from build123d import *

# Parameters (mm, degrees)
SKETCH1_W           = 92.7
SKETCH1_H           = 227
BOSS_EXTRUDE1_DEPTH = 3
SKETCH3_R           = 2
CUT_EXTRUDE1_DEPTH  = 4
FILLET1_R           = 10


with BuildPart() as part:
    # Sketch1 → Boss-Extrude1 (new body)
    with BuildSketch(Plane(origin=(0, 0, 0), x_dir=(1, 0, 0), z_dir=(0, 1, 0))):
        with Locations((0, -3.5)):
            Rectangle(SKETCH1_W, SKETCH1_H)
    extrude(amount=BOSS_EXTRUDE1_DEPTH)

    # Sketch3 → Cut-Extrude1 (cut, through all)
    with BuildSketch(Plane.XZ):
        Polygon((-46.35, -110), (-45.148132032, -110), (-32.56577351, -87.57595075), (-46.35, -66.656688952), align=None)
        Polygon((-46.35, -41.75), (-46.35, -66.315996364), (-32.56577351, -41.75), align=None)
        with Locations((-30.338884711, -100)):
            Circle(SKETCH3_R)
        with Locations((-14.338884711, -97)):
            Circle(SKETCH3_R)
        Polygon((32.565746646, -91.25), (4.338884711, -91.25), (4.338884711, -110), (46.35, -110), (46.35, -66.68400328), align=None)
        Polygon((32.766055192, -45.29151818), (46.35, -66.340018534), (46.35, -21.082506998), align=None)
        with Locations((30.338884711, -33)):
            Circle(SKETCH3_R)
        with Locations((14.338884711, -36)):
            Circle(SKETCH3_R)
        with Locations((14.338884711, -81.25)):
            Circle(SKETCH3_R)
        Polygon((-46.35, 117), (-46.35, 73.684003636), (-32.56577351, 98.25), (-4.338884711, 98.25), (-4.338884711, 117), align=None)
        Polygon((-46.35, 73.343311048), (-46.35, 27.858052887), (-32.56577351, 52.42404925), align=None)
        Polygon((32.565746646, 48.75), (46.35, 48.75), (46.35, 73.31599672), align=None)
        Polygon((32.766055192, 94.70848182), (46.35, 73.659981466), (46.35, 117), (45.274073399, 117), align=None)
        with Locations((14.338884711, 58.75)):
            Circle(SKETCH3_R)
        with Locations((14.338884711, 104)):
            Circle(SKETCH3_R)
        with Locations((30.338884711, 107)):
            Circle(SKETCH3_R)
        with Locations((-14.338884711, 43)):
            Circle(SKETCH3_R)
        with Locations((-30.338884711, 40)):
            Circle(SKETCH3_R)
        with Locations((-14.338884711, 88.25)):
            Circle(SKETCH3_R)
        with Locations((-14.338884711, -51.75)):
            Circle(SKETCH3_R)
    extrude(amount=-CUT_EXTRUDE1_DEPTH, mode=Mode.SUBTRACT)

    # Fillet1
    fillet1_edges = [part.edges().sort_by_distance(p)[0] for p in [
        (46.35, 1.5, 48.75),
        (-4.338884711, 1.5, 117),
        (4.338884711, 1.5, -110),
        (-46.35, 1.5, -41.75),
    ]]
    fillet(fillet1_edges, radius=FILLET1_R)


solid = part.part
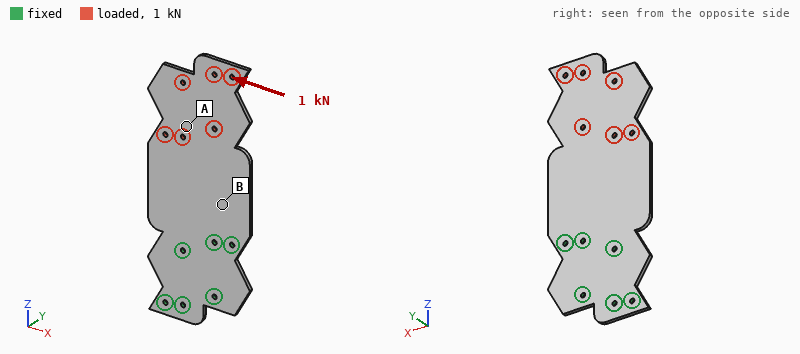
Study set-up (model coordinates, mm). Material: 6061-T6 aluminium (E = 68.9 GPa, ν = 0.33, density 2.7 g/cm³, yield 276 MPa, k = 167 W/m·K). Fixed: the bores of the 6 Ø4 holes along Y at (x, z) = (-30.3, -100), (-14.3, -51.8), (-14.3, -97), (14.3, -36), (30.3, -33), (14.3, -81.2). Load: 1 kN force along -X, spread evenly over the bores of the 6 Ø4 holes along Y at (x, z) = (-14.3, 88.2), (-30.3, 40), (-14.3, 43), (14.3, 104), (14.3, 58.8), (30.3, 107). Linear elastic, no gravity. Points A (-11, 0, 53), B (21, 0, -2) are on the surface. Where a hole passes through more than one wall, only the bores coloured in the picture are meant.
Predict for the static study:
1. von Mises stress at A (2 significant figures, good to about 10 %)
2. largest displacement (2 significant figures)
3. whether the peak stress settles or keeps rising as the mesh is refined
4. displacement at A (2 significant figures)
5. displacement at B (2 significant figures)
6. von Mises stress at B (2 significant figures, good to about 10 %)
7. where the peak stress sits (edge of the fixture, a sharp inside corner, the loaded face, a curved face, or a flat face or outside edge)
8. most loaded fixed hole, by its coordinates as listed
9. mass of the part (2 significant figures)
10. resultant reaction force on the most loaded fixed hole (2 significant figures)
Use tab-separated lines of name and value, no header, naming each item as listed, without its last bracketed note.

von Mises stress at A	6.2 MPa
largest displacement	0.14 mm
whether the peak stress settles or keeps rising as the mesh is refined	keeps rising
displacement at A	0.070 mm
displacement at B	0.024 mm
von Mises stress at B	14 MPa
where the peak stress sits	edge of the fixture
most loaded fixed hole, by its coordinates as listed	(30.3, -33)
mass of the part	140 g
resultant reaction force on the most loaded fixed hole	1.9 kN
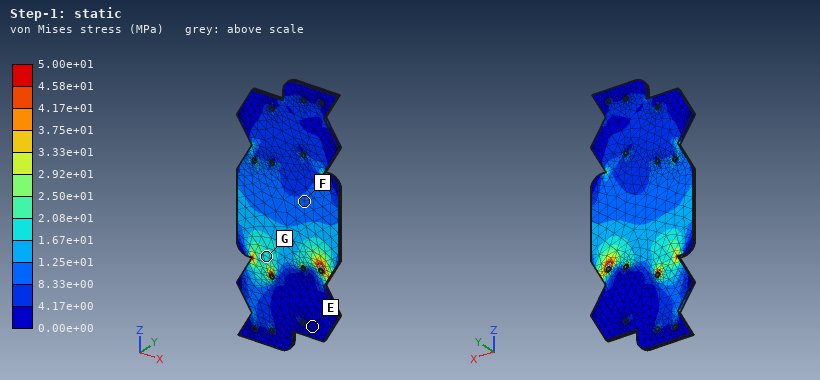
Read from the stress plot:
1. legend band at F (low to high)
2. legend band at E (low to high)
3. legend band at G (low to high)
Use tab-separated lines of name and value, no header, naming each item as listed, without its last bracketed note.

legend band at F	8.33e+00 to 1.25e+01 MPa
legend band at E	0.00e+00 to 4.17e+00 MPa
legend band at G	1.67e+01 to 2.08e+01 MPa
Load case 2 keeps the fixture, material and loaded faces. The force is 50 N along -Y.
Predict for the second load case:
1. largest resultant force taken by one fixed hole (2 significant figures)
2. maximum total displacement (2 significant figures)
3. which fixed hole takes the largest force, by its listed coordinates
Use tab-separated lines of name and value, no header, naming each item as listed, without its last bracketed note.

largest resultant force taken by one fixed hole	98 N
maximum total displacement	2.8 mm
which fixed hole takes the largest force, by its listed coordinates	(14.3, -36)
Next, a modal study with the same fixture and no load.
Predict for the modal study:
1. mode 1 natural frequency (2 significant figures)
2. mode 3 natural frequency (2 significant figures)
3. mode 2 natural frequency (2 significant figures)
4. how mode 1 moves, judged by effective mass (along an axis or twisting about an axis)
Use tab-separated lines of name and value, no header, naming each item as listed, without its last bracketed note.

mode 1 natural frequency	120 Hz
mode 3 natural frequency	690 Hz
mode 2 natural frequency	410 Hz
how mode 1 moves, judged by effective mass	along Y
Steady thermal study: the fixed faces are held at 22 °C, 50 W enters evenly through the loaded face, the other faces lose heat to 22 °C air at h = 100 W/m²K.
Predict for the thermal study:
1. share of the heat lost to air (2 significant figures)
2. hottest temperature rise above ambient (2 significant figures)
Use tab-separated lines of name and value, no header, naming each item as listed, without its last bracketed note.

share of the heat lost to air	88 %
hottest temperature rise above ambient	43 K
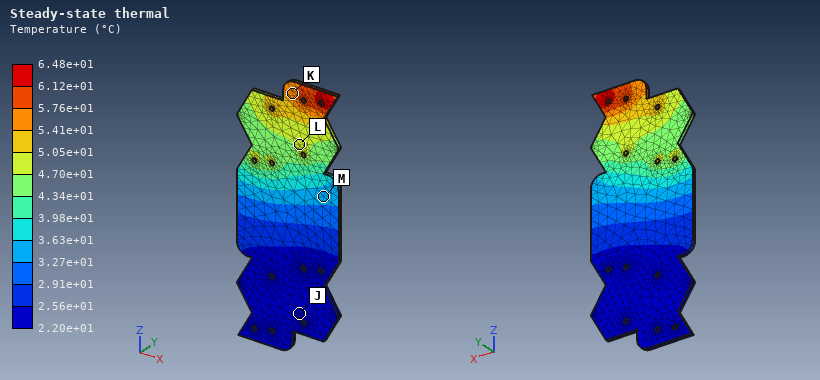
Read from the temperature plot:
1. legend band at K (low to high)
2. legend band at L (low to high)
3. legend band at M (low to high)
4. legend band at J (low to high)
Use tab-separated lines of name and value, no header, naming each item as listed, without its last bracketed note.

legend band at K	5.41e+01 to 5.76e+01 °C
legend band at L	4.70e+01 to 5.05e+01 °C
legend band at M	3.27e+01 to 3.63e+01 °C
legend band at J	2.20e+01 to 2.56e+01 °C
